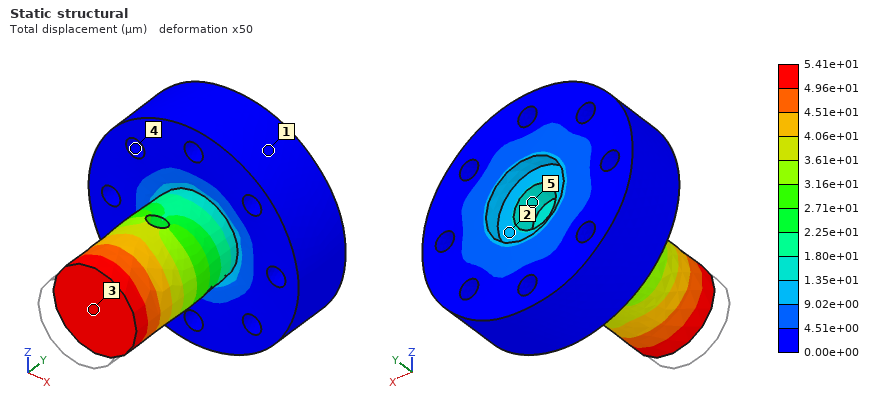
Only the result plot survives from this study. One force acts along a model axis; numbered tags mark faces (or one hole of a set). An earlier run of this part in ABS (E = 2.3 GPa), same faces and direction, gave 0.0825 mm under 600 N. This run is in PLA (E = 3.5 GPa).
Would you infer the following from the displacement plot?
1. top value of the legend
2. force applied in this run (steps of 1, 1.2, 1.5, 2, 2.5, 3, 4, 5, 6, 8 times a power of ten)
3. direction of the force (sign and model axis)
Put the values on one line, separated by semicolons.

5.41e+01 µm; 600 N; +Y
